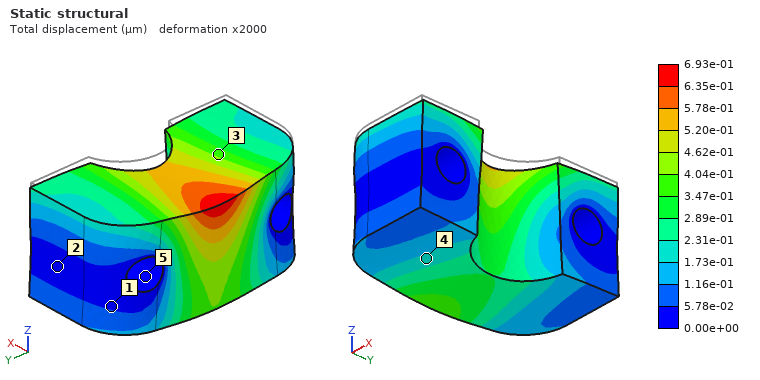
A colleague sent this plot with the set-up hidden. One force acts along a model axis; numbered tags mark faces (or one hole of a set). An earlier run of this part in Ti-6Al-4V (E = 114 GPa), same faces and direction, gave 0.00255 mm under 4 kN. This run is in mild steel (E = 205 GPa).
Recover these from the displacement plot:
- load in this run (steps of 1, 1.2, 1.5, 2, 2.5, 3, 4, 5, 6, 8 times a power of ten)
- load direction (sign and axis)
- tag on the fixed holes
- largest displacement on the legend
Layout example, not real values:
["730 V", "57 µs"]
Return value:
["2 kN", "-Z", "5", "6.93e-01 µm"]
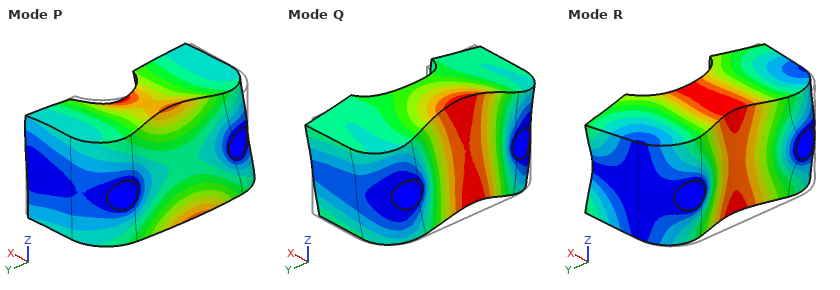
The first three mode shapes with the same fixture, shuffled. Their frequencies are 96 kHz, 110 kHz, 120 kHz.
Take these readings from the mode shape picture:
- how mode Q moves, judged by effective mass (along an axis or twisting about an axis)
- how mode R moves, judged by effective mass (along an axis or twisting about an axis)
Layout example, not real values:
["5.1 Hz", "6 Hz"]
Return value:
["along Z", "along X"]
